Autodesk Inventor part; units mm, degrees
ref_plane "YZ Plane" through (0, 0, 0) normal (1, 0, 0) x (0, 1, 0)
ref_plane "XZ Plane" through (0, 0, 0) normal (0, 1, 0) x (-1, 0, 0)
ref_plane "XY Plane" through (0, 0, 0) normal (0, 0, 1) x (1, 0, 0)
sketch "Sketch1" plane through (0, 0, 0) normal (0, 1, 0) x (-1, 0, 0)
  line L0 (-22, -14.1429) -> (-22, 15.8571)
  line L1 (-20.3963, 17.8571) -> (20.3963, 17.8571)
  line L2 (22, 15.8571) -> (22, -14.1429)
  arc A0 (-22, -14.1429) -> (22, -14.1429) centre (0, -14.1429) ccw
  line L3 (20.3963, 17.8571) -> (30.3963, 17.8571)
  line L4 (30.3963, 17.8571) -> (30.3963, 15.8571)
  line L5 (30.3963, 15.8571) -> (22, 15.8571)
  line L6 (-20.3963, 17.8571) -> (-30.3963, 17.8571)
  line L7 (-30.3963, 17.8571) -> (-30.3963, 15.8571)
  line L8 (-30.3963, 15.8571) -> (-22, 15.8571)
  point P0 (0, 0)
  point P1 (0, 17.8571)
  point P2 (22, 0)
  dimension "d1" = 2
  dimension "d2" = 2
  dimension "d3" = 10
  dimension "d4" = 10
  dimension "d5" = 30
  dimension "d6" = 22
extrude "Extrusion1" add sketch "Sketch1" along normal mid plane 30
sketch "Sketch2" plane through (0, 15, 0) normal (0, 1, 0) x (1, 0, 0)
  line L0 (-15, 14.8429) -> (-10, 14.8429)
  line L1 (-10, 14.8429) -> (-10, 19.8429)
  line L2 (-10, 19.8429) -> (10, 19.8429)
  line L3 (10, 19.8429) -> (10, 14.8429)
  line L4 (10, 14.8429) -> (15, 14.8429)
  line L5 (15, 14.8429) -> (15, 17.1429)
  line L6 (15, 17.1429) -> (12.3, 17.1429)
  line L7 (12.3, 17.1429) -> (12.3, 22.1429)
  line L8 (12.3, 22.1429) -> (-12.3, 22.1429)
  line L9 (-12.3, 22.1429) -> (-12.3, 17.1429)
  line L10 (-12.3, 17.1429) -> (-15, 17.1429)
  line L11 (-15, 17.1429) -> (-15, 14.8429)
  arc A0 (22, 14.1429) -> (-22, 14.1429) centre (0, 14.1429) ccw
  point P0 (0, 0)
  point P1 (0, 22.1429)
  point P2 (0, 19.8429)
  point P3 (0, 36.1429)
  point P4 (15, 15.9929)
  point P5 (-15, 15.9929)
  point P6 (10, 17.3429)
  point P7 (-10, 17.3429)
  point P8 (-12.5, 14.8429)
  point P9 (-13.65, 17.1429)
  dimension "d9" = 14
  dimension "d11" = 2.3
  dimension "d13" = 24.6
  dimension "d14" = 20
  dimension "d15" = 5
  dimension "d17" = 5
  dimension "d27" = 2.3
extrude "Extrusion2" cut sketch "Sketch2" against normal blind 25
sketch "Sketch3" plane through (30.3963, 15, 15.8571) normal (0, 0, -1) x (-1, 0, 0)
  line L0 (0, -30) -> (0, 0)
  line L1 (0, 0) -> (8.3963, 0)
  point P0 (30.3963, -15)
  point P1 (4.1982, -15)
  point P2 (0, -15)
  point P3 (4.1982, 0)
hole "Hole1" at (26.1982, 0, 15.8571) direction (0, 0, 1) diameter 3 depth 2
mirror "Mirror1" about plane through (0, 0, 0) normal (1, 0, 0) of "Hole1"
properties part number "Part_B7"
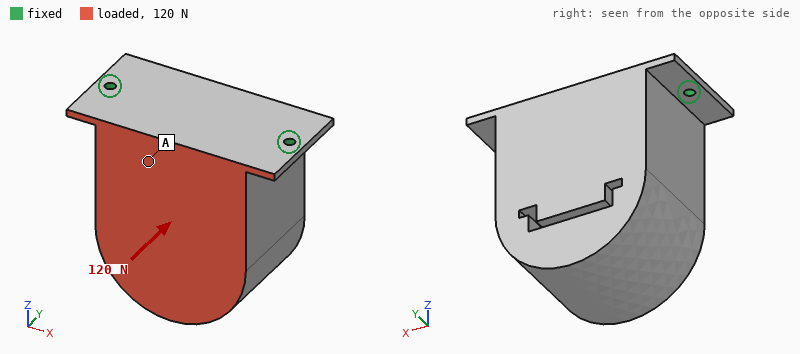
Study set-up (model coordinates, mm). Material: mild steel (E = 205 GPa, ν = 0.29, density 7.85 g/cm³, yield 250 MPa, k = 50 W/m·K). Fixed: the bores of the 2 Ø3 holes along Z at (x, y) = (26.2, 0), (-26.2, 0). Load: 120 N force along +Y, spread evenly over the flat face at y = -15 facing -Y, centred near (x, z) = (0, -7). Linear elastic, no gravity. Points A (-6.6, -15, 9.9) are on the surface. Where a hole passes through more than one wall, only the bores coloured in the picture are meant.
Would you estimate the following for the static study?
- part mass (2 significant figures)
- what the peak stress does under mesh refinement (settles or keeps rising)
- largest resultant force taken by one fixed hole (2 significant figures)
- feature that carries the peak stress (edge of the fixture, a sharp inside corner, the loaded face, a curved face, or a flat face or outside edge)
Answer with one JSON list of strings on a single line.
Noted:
["500 g", "keeps rising", "60 N", "edge of the fixture"]
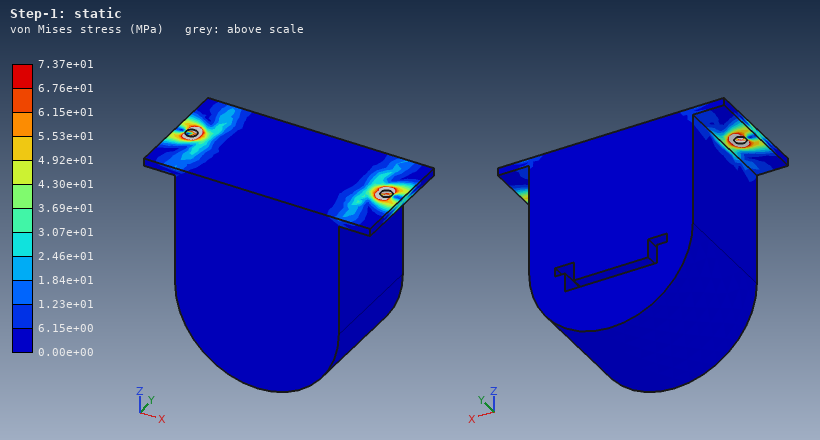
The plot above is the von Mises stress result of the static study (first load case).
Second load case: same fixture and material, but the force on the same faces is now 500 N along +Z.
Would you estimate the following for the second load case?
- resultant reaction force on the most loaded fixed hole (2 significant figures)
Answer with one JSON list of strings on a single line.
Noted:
["280 N"]
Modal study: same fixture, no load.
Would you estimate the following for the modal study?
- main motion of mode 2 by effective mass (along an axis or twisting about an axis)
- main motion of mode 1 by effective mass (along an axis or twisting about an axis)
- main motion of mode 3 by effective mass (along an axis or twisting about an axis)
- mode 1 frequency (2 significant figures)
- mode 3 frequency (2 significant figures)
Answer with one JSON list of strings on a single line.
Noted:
["along X", "along Y", "along Z", "370 Hz", "3300 Hz"]
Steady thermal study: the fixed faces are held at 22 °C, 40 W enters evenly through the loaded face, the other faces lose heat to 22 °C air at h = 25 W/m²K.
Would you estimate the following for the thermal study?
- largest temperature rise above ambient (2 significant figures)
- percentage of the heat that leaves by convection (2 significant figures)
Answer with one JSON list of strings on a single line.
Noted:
["67 K", "37 %"]
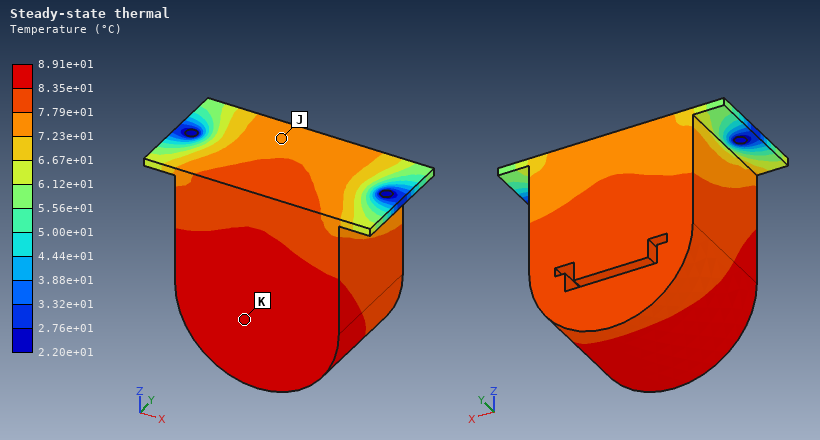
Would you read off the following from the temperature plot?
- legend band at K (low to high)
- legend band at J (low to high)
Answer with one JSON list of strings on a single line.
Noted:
["8.35e+01 to 8.91e+01 °C", "7.23e+01 to 7.79e+01 °C"]
